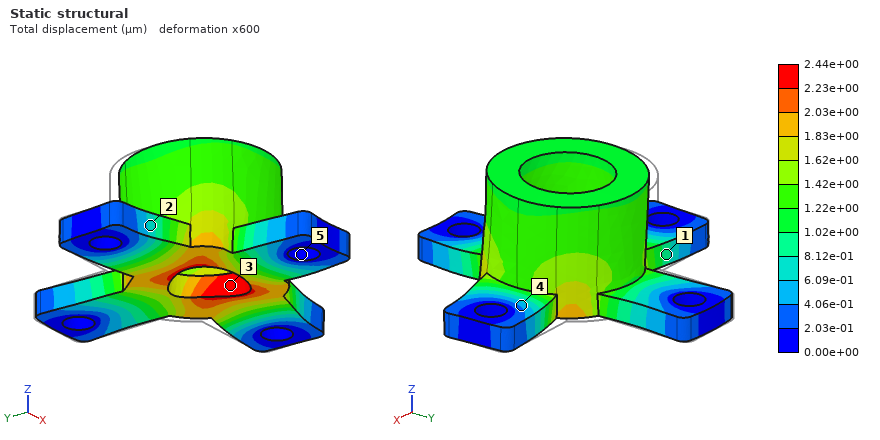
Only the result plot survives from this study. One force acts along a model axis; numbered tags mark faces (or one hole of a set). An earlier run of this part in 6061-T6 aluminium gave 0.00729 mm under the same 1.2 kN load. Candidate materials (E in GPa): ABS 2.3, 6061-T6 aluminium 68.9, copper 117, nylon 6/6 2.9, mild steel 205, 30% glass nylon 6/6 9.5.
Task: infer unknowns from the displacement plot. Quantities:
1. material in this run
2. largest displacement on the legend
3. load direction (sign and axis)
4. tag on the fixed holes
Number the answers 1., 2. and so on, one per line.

1. mild steel
2. 2.44e+00 µm
3. -Y
4. 5
